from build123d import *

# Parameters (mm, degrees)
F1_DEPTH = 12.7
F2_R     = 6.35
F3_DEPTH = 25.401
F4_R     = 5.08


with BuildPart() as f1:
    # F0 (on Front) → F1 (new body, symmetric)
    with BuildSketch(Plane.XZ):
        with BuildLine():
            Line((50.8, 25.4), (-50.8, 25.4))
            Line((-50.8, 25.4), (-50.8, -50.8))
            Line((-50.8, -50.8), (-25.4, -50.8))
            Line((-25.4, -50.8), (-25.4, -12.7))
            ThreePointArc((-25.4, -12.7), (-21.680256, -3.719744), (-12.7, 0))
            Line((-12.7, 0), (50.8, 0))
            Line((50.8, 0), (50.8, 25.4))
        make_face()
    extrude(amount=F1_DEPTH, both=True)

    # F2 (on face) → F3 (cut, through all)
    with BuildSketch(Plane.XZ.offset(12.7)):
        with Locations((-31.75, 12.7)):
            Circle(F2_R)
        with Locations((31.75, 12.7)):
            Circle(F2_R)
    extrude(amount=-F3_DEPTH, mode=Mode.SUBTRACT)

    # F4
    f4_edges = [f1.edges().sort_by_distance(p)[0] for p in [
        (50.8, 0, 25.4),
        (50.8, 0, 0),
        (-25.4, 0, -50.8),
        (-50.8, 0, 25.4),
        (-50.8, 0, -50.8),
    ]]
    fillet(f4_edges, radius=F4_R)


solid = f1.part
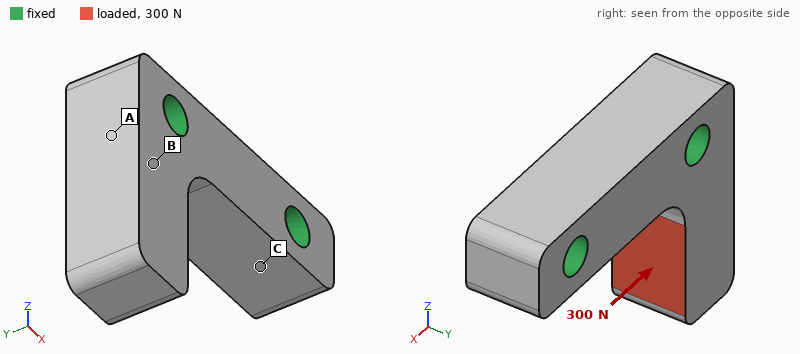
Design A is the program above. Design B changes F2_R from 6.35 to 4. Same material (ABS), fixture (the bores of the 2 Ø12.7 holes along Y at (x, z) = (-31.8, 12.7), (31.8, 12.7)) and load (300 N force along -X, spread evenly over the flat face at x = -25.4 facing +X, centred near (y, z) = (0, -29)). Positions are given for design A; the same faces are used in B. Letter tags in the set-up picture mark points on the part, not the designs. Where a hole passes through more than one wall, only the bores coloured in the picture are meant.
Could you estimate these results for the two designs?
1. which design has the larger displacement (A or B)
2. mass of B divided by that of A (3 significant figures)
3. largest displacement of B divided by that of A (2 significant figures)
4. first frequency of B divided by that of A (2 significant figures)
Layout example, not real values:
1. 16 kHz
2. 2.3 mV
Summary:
1. B
2. 1.04
3. 1.3
4. 0.87
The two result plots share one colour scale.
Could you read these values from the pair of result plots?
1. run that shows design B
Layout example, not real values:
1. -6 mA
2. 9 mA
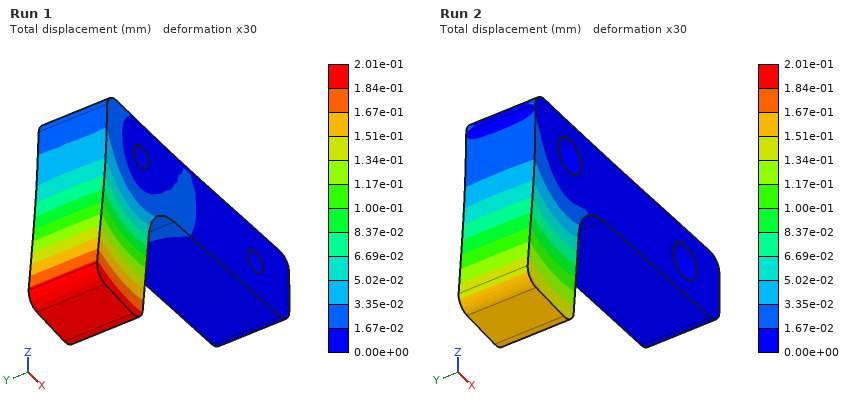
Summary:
1. Run 1
